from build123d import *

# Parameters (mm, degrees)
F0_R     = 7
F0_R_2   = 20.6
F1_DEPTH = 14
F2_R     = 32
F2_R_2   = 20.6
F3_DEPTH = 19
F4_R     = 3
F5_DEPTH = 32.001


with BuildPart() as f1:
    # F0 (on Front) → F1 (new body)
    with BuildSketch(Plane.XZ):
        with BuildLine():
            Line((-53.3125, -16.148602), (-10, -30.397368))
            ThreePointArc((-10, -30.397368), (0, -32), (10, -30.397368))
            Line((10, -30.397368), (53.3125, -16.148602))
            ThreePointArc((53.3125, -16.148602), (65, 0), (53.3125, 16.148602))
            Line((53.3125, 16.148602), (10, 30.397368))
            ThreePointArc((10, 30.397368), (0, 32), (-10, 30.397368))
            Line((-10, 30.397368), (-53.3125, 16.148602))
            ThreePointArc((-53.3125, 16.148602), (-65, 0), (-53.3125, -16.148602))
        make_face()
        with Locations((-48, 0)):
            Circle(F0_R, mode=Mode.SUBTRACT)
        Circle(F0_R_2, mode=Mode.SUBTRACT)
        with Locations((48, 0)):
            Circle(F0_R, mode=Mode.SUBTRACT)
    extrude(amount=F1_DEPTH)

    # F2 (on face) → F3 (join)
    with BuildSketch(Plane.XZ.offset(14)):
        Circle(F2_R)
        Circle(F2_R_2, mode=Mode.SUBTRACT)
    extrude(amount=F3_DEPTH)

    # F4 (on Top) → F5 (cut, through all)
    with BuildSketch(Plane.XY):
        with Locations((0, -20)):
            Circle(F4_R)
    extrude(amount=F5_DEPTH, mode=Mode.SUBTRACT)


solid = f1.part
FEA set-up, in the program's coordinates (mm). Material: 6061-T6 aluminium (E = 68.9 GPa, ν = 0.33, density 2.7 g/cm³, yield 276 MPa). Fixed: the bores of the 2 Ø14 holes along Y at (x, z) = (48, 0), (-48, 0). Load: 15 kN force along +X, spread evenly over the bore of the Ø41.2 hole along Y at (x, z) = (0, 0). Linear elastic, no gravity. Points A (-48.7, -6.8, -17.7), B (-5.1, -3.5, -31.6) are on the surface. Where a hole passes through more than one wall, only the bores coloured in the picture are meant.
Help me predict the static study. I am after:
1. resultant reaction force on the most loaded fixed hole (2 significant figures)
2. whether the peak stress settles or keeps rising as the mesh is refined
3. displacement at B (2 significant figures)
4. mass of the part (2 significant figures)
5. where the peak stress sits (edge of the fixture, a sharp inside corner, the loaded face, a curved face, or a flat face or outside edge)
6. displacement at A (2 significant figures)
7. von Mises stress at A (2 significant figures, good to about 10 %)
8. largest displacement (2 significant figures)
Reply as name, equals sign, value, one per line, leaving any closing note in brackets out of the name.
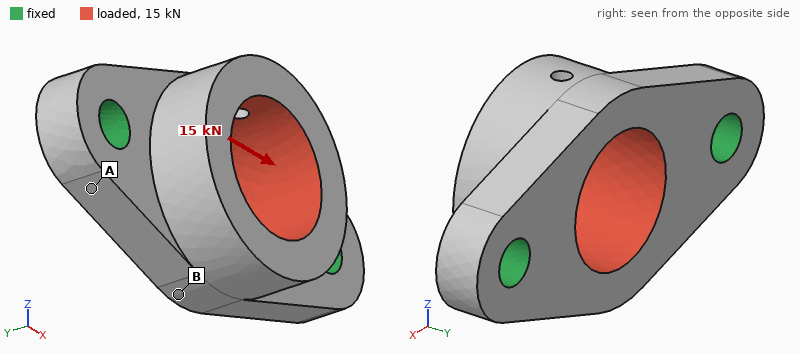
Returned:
resultant reaction force on the most loaded fixed hole = 7.7 kN
whether the peak stress settles or keeps rising as the mesh is refined = keeps rising
displacement at B = 6.4 µm
mass of the part = 250 g
where the peak stress sits = edge of the fixture
displacement at A = 2.8 µm
von Mises stress at A = 8.1 MPa
largest displacement = 13 µm
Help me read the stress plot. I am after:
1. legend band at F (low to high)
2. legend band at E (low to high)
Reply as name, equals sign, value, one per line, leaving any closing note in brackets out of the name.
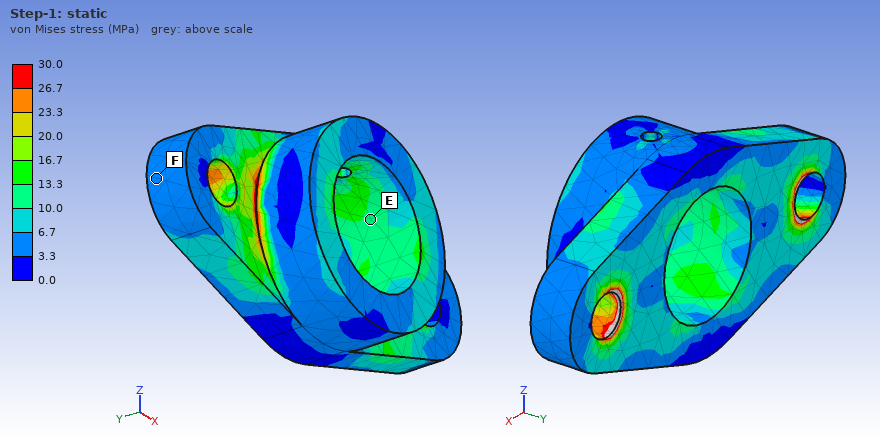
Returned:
legend band at F = 3.3 to 6.7 MPa
legend band at E = 10.0 to 13.3 MPa
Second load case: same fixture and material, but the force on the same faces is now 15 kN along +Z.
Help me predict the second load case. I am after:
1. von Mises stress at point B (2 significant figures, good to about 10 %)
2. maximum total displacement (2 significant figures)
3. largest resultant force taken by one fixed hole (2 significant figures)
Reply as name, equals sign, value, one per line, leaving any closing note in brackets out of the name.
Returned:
von Mises stress at point B = 16 MPa
maximum total displacement = 77 µm
largest resultant force taken by one fixed hole = 7.5 kN
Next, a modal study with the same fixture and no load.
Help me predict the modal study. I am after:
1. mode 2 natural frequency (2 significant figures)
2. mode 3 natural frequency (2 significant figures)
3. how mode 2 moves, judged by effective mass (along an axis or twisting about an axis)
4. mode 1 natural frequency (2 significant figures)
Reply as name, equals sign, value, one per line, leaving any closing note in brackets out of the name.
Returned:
mode 2 natural frequency = 7100 Hz
mode 3 natural frequency = 12 kHz
how mode 2 moves, judged by effective mass = along Y
mode 1 natural frequency = 4900 Hz
